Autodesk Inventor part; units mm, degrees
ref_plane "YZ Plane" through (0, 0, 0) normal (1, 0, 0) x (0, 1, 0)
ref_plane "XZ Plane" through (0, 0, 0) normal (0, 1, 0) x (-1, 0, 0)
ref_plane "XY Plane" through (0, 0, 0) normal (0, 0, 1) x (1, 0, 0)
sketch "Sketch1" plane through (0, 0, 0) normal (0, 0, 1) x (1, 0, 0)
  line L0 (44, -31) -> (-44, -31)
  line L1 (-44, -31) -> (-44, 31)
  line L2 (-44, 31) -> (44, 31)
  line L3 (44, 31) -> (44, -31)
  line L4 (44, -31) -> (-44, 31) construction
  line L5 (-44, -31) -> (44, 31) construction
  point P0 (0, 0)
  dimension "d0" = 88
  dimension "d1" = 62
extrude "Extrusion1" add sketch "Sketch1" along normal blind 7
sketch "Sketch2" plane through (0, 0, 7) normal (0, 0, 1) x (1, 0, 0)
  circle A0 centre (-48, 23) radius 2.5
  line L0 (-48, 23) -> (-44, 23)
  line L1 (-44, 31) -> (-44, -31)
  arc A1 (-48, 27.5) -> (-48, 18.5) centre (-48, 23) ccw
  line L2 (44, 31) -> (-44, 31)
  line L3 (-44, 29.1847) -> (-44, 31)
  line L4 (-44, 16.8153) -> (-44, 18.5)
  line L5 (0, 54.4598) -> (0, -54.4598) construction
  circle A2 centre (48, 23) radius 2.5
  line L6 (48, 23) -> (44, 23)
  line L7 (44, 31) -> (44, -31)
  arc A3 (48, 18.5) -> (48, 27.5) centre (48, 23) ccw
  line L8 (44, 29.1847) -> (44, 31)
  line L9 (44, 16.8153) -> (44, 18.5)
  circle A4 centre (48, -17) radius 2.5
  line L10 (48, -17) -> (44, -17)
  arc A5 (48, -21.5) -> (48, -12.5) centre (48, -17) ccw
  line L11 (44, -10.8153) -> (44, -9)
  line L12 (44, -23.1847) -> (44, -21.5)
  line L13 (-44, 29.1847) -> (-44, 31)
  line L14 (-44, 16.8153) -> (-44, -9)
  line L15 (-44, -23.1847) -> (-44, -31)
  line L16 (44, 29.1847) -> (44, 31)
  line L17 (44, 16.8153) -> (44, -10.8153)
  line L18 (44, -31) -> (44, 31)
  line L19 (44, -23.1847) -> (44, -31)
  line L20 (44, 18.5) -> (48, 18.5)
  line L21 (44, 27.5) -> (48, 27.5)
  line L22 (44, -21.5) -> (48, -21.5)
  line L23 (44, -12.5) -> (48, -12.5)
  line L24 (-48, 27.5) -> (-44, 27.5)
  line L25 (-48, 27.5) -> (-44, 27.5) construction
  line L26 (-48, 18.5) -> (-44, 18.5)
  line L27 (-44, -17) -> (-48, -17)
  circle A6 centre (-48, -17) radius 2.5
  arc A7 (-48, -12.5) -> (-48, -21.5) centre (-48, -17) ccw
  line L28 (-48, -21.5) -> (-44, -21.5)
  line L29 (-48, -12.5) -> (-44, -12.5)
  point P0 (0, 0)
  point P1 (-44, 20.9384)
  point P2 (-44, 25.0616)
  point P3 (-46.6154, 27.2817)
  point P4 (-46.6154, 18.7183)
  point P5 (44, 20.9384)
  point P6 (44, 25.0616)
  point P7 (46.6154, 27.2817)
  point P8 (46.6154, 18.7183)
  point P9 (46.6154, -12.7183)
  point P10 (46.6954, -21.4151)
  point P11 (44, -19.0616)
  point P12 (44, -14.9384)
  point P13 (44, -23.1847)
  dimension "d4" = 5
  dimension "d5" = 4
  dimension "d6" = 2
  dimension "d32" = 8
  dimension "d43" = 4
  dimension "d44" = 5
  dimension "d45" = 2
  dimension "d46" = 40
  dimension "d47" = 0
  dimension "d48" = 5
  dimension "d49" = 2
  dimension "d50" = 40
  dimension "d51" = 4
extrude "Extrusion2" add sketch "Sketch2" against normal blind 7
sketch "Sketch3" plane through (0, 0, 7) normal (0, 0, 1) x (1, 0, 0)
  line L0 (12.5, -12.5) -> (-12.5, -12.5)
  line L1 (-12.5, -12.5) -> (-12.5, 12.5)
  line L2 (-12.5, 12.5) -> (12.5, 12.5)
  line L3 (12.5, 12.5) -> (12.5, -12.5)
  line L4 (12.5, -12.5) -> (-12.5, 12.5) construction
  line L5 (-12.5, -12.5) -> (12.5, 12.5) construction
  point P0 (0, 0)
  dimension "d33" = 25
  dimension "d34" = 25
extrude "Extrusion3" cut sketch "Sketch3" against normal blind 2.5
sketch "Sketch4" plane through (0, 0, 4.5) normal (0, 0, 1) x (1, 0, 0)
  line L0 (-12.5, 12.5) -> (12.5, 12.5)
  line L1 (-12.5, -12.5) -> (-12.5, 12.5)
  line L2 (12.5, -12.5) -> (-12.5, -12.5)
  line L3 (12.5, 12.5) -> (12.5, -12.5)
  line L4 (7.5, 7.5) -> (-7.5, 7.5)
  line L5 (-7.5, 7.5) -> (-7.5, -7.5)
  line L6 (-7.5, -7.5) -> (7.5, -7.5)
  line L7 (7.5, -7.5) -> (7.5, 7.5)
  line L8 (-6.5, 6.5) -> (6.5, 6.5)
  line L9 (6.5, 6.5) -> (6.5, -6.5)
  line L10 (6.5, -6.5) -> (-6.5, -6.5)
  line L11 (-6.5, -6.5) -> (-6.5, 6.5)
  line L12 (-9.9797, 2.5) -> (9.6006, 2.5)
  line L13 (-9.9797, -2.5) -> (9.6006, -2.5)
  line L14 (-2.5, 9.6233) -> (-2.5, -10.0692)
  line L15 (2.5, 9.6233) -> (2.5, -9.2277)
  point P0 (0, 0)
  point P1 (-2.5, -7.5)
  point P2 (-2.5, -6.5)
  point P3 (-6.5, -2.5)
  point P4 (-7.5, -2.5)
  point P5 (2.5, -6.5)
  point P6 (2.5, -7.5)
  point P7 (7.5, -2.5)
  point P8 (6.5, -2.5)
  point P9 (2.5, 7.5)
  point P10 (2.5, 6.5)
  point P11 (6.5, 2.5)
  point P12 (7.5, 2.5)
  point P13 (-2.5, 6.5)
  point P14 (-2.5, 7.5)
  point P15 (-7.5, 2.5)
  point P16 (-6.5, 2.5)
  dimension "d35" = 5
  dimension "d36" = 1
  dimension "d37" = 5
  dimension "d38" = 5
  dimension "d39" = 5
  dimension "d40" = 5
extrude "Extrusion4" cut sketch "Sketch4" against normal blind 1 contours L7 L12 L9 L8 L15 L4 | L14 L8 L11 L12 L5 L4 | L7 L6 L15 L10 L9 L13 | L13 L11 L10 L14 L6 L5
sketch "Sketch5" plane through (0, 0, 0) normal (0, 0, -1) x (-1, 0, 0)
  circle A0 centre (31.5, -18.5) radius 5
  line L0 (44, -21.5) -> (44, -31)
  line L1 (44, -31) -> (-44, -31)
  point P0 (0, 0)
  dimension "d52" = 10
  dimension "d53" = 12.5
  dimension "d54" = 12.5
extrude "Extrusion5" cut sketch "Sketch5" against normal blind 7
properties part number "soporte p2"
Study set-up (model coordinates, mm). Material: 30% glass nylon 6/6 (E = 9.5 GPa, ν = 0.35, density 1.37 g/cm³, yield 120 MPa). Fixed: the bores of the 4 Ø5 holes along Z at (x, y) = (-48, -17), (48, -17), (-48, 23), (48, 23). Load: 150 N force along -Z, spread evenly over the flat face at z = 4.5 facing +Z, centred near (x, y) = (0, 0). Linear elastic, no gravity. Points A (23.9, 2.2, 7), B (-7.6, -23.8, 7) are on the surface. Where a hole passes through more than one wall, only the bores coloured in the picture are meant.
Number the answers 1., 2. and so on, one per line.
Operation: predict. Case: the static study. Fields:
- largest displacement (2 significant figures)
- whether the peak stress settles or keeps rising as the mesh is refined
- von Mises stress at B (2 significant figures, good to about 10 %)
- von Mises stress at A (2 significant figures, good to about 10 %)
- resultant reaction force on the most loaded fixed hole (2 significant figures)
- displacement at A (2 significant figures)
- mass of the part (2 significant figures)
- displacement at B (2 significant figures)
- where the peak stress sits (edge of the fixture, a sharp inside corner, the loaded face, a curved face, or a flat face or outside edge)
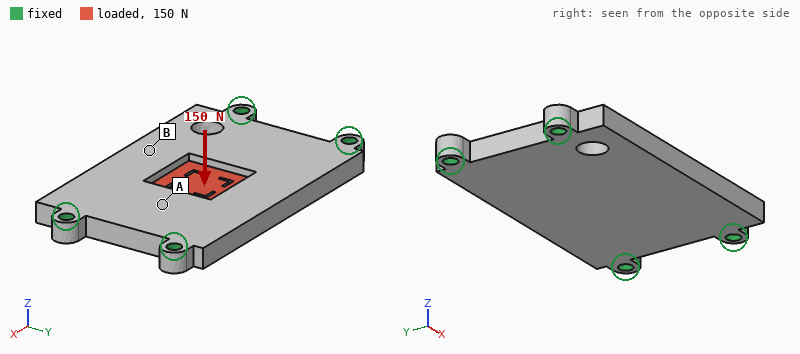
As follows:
1. 76 µm
2. keeps rising
3. 3.5 MPa
4. 1.3 MPa
5. 49 N
6. 41 µm
7. 51 g
8. 59 µm
9. edge of the fixture
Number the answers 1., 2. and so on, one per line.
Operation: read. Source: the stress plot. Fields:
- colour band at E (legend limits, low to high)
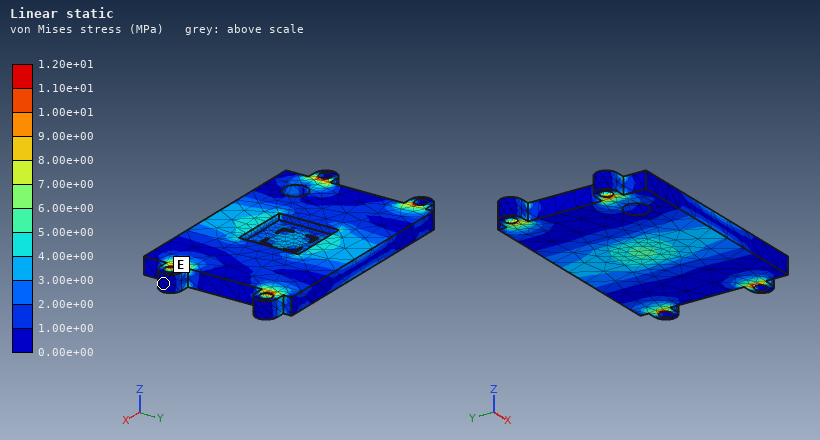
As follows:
1. 0.00e+00 to 1.00e+00 MPa
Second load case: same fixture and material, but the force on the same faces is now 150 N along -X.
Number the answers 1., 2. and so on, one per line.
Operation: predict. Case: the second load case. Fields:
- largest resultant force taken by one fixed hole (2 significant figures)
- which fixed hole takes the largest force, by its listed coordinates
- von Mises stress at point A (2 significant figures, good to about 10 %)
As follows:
1. 44 N
2. (48, -17)
3. 0.19 MPa
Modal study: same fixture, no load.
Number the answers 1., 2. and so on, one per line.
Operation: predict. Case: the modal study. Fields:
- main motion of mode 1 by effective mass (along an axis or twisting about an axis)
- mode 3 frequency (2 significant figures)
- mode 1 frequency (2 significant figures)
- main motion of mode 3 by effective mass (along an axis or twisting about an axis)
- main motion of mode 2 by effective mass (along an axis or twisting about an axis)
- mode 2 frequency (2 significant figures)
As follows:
1. along Z
2. 4500 Hz
3. 1600 Hz
4. twisting about Y
5. twisting about X
6. 2500 Hz
